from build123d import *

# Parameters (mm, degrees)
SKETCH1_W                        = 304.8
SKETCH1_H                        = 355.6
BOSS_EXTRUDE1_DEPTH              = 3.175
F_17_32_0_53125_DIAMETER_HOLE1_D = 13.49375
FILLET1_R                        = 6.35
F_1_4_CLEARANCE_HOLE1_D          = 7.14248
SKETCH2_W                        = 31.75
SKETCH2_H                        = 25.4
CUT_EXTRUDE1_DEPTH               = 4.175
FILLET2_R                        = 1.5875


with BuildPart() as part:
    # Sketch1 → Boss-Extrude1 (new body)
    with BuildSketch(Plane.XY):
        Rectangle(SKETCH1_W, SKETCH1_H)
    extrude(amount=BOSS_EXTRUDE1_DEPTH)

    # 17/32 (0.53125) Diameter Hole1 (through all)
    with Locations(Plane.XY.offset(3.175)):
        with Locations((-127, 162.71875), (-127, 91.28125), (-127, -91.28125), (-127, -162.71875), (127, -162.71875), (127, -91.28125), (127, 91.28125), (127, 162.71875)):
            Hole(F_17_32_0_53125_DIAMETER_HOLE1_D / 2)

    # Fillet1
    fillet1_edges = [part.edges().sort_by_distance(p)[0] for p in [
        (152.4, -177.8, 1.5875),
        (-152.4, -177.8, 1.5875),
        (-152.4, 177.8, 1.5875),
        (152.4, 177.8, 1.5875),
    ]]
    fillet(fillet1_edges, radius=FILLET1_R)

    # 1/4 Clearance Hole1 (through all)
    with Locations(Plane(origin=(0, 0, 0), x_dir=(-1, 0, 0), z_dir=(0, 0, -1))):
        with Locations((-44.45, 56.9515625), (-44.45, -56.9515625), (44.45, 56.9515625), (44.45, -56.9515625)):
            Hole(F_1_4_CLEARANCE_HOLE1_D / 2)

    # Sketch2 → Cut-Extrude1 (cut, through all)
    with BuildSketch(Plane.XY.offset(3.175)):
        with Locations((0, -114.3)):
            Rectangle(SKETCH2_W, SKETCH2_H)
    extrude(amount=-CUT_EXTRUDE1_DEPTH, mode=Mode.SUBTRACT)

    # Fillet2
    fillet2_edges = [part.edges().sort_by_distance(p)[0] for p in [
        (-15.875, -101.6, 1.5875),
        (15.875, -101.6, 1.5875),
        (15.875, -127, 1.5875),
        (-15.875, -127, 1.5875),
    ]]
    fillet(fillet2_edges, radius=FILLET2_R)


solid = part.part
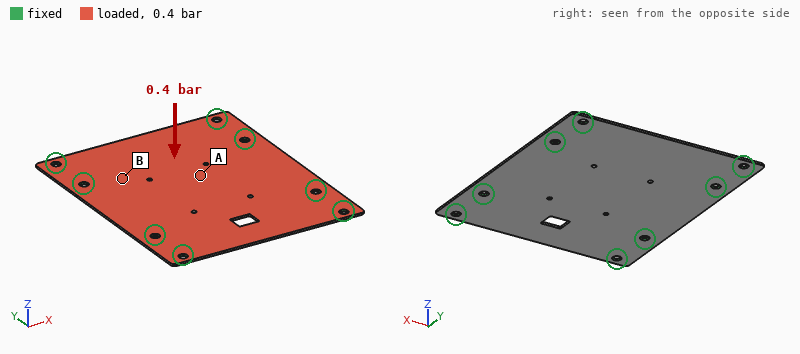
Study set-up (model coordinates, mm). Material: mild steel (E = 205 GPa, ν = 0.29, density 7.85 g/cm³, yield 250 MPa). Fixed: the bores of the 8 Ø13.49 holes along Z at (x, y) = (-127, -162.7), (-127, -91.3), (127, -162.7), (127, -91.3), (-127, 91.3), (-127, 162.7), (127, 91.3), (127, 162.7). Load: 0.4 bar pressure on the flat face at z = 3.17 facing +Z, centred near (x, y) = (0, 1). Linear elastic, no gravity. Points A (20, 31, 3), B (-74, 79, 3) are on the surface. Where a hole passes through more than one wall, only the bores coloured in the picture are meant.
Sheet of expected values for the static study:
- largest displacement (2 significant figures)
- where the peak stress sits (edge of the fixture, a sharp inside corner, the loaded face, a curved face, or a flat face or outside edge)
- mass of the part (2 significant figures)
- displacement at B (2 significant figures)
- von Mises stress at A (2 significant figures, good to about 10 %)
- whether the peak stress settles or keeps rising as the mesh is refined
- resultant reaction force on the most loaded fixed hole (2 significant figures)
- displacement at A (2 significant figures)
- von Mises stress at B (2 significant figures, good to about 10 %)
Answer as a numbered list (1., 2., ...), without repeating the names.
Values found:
1. 1.1 mm
2. edge of the fixture
3. 2.6 kg
4. 0.45 mm
5. 56 MPa
6. keeps rising
7. 810 N
8. 1.0 mm
9. 25 MPa
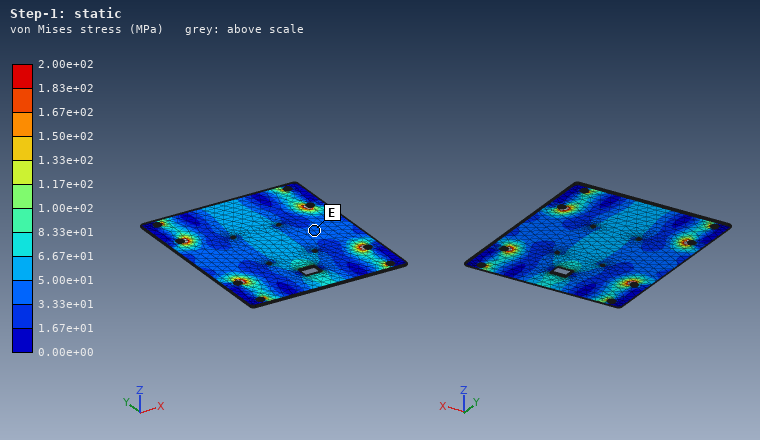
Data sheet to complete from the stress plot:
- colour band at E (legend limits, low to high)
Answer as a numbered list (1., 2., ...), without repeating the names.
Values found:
1. 3.33e+01 to 5.00e+01 MPa
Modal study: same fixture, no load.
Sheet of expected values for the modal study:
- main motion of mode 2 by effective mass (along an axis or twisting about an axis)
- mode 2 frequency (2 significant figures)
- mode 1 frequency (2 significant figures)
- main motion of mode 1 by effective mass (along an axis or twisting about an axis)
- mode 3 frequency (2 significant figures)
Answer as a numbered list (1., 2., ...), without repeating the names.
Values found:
1. twisting about X
2. 300 Hz
3. 240 Hz
4. along Z
5. 370 Hz
